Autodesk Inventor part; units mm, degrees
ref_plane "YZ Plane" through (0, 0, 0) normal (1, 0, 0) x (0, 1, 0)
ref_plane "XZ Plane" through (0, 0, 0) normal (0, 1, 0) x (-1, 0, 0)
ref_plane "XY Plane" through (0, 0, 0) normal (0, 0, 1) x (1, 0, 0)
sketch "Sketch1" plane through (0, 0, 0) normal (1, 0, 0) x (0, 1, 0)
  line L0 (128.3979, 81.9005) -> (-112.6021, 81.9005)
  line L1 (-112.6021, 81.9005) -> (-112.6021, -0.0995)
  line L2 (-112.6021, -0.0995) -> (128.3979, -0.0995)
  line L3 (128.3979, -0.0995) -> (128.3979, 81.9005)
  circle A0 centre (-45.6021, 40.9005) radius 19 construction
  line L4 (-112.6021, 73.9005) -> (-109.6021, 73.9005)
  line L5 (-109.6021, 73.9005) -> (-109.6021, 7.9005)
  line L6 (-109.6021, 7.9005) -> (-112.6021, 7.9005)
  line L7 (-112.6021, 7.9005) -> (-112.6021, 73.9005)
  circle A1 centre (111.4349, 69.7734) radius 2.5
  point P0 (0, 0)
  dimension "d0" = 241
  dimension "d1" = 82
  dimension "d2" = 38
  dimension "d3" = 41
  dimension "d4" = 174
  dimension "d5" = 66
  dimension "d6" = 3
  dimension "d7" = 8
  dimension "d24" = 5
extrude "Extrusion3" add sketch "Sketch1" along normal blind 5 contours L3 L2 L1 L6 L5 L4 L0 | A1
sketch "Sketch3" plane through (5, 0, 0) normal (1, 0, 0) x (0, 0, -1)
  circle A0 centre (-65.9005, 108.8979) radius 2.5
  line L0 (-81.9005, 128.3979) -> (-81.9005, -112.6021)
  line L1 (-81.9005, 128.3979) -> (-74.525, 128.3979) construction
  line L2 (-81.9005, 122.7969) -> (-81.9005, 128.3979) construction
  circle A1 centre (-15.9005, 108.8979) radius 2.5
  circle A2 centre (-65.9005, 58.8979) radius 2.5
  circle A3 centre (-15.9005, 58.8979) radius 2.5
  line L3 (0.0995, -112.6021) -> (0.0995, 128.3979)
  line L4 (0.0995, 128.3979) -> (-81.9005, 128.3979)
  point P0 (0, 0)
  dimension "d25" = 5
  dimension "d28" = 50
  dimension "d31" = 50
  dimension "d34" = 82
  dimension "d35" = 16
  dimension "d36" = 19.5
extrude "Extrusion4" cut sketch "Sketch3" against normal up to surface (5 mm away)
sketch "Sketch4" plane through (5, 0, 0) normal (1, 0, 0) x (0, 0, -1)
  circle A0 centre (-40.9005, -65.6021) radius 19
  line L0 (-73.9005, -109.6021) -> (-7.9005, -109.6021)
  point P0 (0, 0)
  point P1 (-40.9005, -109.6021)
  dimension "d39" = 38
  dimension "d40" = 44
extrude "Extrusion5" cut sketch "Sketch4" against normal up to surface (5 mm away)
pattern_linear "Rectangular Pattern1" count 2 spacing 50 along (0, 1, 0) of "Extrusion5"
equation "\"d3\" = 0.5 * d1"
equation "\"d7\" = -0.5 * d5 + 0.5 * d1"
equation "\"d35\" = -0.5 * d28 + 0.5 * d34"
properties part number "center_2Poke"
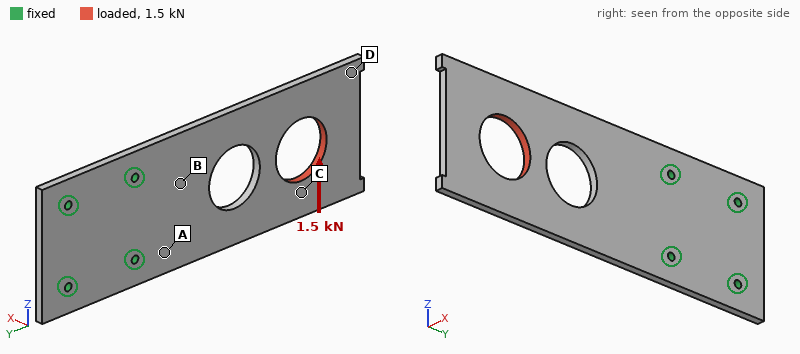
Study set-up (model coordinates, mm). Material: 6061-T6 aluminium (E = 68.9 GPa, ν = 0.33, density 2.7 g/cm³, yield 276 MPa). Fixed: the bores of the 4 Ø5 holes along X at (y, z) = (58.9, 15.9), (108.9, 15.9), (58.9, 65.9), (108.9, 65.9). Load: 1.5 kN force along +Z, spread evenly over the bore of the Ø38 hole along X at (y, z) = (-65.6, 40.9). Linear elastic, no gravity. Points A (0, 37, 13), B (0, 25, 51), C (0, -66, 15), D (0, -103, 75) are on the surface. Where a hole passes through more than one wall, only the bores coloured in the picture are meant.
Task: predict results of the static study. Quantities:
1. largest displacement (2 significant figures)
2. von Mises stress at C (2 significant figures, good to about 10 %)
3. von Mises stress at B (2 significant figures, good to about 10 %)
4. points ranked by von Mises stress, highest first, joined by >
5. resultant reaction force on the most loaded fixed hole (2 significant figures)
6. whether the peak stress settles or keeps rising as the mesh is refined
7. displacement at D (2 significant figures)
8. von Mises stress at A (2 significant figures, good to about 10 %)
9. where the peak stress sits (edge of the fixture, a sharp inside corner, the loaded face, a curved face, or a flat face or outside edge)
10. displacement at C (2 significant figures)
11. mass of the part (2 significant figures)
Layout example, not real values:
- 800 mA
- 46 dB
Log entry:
- 0.19 mm
- 9.3 MPa
- 13 MPa
- A > B > C > D
- 2.9 kN
- keeps rising
- 0.18 mm
- 20 MPa
- edge of the fixture
- 0.14 mm
- 230 g
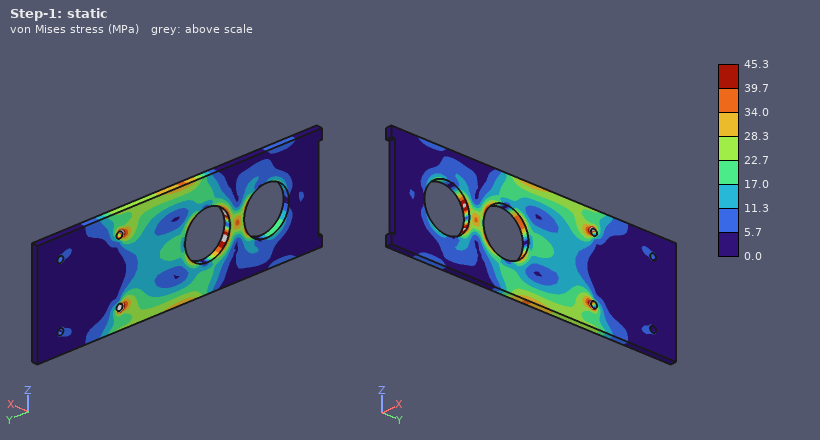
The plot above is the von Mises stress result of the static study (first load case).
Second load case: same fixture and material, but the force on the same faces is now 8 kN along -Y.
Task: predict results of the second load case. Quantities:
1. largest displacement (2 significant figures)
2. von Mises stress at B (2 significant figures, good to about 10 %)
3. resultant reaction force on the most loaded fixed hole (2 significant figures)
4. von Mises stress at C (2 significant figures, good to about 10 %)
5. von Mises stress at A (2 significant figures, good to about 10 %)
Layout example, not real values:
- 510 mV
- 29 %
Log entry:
- 67 µm
- 13 MPa
- 3.3 kN
- 24 MPa
- 25 MPa
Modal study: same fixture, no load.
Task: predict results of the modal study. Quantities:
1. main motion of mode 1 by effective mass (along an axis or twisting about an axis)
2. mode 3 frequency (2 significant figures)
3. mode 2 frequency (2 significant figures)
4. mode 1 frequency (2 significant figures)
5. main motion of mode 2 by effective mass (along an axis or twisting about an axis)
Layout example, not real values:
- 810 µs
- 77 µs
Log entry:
- along X
- 830 Hz
- 550 Hz
- 140 Hz
- twisting about Y
